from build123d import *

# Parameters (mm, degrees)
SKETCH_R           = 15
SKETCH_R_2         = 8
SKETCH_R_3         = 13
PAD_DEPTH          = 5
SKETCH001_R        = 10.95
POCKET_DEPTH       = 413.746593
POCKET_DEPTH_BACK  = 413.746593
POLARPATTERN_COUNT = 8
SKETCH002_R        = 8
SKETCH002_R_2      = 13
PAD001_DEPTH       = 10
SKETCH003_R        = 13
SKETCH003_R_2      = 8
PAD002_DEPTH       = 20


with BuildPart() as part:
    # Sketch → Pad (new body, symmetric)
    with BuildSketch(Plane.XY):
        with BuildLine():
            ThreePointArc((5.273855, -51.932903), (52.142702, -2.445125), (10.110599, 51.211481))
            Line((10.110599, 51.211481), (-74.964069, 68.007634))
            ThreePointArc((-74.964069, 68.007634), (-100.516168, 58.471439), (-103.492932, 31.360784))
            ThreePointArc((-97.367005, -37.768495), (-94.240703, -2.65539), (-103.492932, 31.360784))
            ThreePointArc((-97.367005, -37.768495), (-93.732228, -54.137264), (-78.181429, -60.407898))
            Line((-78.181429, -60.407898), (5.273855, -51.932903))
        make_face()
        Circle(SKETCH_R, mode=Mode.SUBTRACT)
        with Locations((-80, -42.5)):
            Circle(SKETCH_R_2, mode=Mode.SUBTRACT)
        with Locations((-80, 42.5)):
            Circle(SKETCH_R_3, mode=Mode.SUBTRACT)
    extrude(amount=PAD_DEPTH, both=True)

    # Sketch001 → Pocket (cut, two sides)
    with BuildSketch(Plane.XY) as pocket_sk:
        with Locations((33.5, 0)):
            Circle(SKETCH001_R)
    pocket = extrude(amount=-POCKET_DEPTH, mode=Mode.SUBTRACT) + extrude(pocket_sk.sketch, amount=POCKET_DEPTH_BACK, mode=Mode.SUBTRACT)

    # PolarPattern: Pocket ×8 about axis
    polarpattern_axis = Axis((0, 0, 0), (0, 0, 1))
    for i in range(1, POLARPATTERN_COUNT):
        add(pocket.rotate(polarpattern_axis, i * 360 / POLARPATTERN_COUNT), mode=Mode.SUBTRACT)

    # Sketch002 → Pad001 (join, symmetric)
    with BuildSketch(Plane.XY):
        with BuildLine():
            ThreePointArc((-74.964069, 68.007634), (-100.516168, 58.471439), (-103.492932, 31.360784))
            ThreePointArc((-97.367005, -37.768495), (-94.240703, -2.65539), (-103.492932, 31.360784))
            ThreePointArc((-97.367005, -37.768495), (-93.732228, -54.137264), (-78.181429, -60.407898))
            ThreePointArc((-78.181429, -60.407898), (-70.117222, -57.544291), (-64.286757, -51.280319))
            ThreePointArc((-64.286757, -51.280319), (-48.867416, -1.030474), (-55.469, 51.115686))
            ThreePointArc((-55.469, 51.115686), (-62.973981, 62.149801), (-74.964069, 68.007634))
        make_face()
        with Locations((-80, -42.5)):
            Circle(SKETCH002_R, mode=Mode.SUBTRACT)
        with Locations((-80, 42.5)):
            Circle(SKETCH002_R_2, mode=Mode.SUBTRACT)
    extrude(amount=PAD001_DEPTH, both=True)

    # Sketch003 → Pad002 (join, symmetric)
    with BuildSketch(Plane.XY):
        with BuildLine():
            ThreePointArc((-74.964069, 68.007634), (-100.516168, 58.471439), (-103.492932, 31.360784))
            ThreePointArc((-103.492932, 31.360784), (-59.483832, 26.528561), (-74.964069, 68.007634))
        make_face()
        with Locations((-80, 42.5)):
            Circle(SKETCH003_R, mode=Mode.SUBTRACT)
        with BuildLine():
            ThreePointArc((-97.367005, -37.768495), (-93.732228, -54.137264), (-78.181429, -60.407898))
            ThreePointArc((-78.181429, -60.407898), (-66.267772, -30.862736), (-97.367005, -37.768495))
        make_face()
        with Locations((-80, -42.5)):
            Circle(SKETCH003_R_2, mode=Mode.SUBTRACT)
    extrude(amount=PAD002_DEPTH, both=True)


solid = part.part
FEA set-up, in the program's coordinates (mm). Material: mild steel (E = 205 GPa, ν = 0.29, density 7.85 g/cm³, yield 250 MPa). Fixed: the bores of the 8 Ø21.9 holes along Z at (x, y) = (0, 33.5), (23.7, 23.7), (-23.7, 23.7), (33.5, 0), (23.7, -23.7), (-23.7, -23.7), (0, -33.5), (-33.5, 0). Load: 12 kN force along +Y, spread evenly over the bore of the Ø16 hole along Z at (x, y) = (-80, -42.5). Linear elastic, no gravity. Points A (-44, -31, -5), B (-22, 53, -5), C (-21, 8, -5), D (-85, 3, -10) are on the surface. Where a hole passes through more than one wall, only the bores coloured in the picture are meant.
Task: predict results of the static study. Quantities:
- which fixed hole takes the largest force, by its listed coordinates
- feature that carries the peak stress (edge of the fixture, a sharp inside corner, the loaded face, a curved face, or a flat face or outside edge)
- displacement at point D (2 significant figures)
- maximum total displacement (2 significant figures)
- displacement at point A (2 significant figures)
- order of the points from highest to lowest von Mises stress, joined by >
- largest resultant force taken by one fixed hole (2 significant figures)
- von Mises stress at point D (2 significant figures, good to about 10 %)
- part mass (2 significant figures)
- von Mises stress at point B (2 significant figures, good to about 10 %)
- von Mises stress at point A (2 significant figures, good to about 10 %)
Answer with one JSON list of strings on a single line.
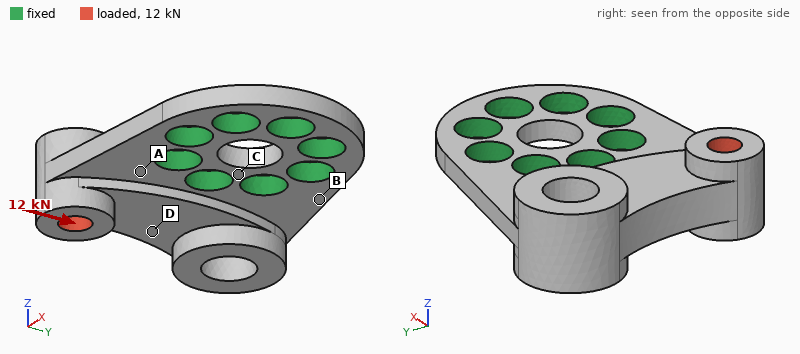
["(-33.5, 0)", "edge of the fixture", "7.6 µm", "14 µm", "2.4 µm", "A > B > D > C", "8.4 kN", "10 MPa", "1.7 kg", "14 MPa", "22 MPa"]
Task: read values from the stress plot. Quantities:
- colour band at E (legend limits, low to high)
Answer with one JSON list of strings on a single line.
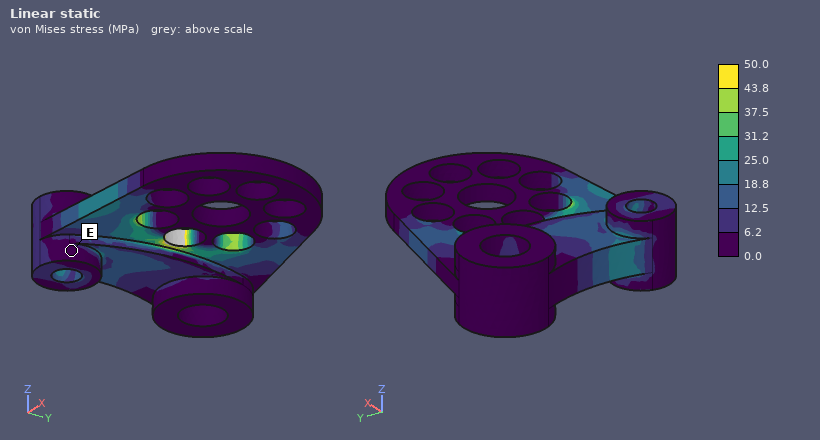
["0.0 to 6.2 MPa"]
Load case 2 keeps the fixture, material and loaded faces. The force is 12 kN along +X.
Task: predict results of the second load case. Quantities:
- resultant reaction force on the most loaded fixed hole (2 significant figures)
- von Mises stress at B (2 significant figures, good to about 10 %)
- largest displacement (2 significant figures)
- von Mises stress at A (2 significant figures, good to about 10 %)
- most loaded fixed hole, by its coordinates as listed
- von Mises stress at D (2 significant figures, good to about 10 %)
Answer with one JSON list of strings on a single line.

["8.4 kN", "6.6 MPa", "12 µm", "32 MPa", "(-23.7, -23.7)", "5.8 MPa"]
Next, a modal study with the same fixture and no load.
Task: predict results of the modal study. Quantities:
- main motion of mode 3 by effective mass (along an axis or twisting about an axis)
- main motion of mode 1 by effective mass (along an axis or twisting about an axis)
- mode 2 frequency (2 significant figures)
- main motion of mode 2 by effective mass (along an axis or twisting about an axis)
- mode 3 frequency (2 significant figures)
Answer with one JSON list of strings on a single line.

["along Y", "along Z", "2400 Hz", "twisting about X", "5400 Hz"]
